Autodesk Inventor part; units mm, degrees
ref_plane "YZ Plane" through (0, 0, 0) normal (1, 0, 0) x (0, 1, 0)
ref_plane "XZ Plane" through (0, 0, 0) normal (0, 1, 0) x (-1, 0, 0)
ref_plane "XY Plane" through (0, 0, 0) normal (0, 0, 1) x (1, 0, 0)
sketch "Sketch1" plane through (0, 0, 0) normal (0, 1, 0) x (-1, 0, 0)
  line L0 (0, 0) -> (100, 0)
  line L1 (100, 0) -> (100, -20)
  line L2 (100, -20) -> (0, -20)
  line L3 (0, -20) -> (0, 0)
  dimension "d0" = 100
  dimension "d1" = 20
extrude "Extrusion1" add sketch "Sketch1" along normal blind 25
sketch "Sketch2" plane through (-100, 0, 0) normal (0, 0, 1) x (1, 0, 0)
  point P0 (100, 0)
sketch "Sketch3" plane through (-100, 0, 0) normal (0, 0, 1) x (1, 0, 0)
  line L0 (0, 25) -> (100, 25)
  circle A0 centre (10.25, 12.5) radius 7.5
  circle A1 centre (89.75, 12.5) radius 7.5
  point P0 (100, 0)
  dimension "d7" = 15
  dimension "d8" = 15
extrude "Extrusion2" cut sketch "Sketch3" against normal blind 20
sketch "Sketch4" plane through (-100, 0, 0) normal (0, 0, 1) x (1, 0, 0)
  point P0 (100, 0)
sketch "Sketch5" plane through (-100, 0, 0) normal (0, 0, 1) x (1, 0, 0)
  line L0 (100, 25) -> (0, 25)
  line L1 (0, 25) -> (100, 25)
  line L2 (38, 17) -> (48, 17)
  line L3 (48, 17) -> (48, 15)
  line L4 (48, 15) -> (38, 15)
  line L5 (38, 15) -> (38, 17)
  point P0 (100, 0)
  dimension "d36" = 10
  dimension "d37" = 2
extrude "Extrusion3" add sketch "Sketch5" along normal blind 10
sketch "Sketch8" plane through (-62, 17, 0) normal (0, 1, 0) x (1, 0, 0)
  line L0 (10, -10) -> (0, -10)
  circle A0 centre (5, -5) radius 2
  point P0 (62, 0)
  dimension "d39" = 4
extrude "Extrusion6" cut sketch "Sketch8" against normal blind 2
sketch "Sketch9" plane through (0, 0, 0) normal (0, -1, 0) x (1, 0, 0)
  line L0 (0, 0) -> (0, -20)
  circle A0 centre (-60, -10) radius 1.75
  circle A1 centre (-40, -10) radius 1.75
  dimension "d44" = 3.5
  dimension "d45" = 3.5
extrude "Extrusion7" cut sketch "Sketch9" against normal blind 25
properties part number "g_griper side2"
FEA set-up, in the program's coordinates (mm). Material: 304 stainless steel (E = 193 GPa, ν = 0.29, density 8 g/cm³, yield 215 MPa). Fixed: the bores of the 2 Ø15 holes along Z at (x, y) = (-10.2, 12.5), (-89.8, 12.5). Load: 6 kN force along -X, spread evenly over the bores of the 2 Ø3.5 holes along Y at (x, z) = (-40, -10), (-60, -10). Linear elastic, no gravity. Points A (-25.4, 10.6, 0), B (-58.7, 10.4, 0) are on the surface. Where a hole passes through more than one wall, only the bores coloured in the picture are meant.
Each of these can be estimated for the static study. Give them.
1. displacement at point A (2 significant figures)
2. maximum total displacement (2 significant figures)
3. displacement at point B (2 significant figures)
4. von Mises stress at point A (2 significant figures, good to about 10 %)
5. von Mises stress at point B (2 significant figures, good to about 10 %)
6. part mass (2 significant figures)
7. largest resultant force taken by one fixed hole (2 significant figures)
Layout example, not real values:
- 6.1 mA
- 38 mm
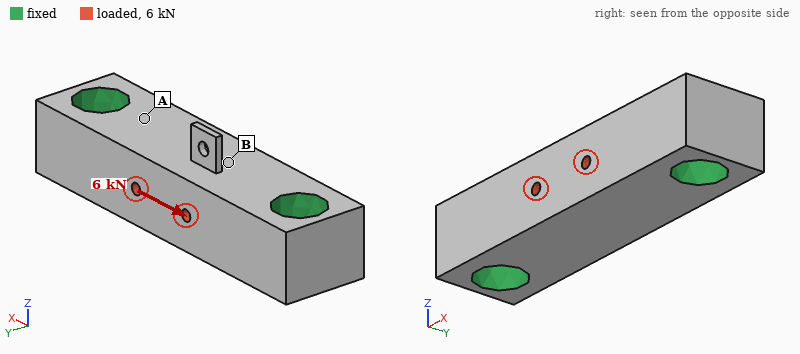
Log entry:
- 0.33 µm
- 1.0 µm
- 0.69 µm
- 6.8 MPa
- 3.0 MPa
- 340 g
- 3.0 kN
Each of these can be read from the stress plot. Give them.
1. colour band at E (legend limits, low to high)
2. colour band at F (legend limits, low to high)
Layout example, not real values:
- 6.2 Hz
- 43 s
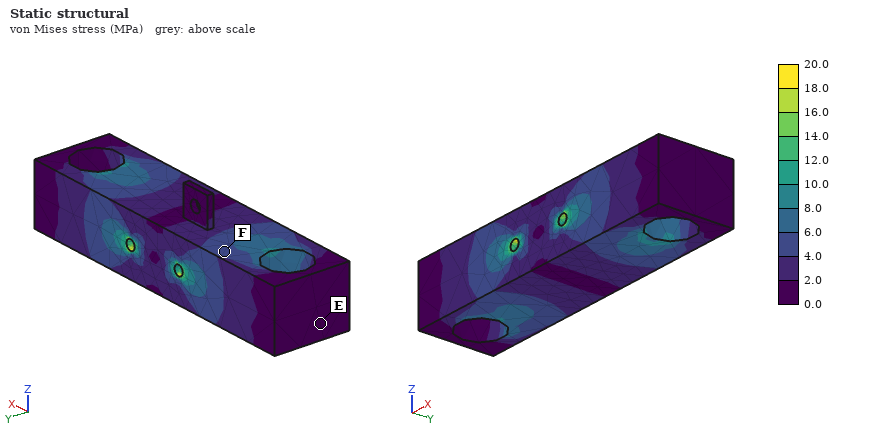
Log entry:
- 0.0 to 2.0 MPa
- 4.0 to 6.0 MPa
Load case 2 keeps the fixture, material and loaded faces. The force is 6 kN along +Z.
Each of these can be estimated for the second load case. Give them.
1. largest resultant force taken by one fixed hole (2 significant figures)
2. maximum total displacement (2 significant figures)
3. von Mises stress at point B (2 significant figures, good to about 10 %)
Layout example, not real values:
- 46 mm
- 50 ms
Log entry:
- 3.0 kN
- 5.1 µm
- 17 MPa
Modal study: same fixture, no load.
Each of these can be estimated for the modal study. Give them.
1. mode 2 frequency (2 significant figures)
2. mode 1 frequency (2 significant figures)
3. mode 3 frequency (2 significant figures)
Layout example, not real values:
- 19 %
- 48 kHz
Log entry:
- 15 kHz
- 13 kHz
- 15 kHz
